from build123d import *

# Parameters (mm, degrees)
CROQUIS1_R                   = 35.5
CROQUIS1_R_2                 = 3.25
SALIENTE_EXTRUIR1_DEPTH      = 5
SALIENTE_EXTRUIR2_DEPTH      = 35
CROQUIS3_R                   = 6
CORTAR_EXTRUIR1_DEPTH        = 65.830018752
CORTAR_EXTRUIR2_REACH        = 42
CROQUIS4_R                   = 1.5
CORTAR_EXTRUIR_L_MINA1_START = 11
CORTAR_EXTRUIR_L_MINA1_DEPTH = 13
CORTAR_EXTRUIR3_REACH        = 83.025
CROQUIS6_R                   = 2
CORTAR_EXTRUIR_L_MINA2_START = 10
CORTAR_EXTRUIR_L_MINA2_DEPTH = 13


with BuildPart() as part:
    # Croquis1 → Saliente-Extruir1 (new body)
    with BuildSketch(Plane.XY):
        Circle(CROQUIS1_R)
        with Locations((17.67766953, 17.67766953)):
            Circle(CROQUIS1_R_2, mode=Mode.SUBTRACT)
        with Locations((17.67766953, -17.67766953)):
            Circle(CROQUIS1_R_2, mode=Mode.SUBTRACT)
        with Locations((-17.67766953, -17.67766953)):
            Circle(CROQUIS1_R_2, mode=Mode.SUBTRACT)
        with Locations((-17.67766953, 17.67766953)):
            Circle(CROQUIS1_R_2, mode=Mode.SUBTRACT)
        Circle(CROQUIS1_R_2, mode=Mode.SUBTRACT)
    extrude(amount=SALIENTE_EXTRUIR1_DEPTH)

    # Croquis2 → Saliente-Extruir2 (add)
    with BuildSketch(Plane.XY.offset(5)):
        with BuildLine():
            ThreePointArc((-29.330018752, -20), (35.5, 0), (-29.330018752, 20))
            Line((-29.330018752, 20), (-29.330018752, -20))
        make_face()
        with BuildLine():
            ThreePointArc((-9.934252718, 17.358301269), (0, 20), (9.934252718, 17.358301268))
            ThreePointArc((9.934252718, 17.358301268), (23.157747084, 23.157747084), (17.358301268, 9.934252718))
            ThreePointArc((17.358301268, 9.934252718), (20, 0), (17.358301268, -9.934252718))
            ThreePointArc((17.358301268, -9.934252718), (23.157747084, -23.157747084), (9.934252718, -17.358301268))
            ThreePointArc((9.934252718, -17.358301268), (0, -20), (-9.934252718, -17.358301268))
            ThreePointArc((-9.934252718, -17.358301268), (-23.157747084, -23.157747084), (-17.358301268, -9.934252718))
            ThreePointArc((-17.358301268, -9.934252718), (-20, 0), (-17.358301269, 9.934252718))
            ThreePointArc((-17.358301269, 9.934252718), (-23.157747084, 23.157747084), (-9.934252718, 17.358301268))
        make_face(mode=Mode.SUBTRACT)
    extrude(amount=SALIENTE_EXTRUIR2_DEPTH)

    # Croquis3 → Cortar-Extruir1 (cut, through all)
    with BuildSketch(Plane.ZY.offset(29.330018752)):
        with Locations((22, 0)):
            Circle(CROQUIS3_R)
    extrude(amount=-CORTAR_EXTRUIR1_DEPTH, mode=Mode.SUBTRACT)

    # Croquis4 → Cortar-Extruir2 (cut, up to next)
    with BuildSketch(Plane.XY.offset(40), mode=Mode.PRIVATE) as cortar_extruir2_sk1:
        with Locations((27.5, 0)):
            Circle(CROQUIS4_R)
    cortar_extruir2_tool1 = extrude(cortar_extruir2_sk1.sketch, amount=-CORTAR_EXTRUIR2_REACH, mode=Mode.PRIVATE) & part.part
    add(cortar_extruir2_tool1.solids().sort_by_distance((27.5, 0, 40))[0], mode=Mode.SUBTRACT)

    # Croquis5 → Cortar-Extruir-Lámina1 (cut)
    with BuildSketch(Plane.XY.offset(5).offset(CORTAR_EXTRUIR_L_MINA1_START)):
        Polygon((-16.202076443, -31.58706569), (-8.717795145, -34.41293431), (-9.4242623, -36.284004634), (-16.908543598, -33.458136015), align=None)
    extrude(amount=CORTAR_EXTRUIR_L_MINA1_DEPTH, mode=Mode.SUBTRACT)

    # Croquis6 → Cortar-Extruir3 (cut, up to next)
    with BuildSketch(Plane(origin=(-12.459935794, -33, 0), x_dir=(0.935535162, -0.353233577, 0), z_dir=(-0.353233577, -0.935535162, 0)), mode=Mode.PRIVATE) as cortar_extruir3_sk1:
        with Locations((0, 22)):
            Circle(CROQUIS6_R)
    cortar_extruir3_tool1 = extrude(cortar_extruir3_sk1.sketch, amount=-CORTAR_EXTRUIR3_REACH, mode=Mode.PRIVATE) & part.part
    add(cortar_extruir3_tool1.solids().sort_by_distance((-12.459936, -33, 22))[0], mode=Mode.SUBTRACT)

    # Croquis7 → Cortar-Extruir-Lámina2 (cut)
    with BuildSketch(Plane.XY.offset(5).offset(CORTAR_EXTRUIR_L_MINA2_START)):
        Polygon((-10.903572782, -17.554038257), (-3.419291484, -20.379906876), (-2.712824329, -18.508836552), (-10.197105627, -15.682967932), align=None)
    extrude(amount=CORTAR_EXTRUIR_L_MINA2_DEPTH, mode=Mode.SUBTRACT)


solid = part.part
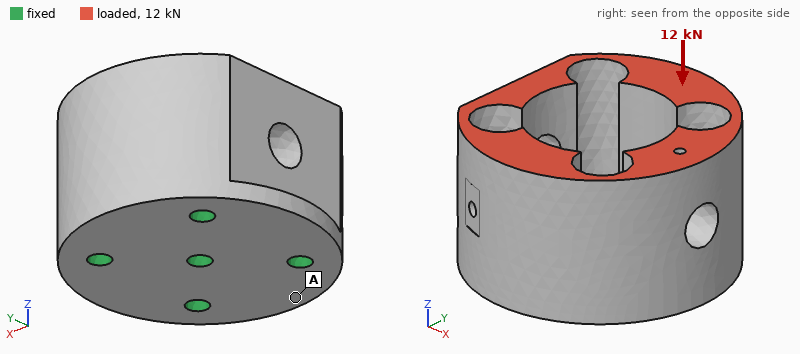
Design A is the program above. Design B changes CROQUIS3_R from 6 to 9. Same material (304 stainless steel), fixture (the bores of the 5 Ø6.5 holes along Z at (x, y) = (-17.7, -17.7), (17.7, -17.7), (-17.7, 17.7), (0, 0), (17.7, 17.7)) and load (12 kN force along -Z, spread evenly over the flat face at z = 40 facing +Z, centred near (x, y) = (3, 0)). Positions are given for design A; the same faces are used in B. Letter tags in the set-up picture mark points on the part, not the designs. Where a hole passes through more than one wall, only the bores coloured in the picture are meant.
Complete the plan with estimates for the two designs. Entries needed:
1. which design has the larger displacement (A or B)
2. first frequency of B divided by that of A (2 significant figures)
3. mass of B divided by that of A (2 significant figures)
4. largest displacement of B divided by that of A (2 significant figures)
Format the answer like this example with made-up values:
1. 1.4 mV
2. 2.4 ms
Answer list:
1. B
2. 0.96
3. 0.95
4. 1.2
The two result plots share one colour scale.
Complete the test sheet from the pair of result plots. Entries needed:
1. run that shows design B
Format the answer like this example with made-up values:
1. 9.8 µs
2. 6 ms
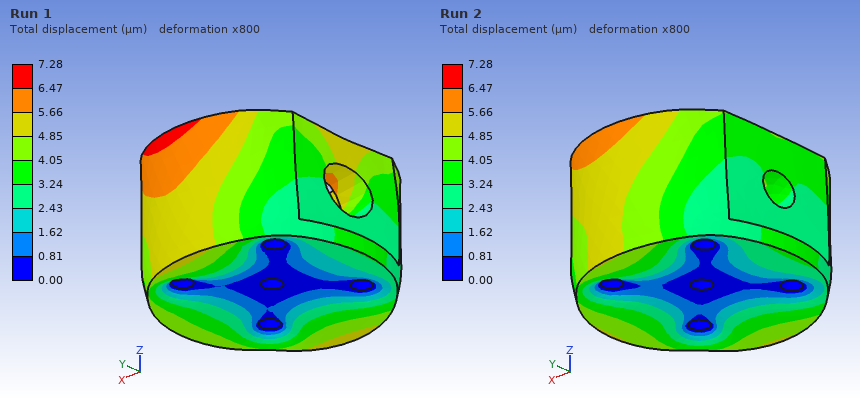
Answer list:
1. Run 1
